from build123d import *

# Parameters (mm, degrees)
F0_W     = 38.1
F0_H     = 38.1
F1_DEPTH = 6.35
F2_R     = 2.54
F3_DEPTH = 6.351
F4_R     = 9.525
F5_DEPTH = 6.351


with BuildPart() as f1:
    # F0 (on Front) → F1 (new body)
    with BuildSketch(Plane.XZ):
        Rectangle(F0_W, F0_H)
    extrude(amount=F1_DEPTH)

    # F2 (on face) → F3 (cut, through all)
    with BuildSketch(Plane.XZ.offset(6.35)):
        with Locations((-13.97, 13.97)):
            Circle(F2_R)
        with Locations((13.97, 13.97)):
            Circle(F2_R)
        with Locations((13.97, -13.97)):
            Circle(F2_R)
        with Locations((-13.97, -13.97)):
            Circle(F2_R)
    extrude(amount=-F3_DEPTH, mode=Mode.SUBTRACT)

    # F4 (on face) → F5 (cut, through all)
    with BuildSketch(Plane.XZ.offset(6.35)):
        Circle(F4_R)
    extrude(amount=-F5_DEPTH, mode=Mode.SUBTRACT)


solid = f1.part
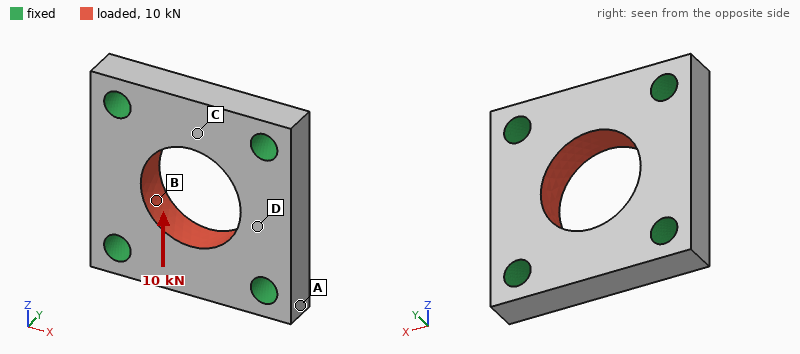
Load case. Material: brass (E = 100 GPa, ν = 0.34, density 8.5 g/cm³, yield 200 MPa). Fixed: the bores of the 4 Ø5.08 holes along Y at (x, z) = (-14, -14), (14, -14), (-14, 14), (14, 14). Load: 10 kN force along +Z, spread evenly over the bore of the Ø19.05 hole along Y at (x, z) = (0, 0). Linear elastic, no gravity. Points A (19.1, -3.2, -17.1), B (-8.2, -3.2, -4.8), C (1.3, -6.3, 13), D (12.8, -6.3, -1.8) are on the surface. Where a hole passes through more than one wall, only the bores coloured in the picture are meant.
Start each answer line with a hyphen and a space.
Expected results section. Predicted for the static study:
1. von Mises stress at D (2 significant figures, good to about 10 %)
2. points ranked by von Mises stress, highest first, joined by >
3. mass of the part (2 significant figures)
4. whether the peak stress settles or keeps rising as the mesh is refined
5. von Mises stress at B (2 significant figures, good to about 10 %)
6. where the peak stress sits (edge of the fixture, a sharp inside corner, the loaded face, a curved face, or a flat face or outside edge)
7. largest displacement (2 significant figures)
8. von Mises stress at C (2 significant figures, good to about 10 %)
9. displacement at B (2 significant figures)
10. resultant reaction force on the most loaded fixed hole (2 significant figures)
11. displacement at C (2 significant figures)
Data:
- 32 MPa
- B > D > C > A
- 59 g
- keeps rising
- 53 MPa
- edge of the fixture
- 8.2 µm
- 19 MPa
- 4.4 µm
- 2.6 kN
- 7.4 µm
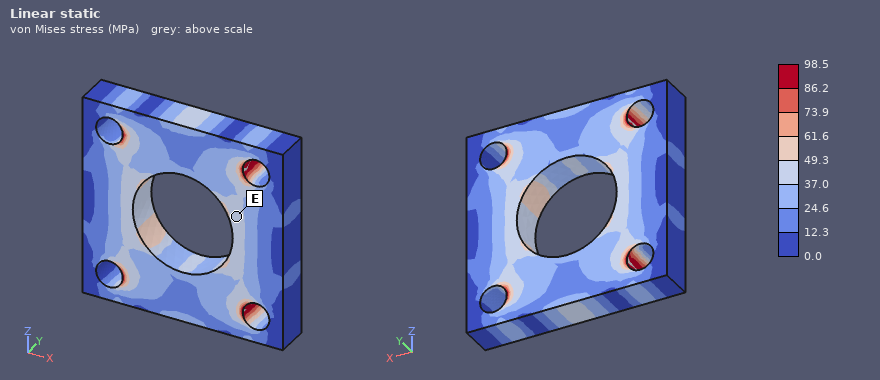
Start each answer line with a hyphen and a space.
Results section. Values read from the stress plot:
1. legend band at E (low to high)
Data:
- 37.0 to 49.3 MPa
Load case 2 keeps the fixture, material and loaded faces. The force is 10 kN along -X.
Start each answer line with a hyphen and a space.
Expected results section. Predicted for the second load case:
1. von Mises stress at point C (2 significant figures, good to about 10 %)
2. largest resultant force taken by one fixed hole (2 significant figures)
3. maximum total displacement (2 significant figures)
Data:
- 31 MPa
- 2.6 kN
- 8.2 µm
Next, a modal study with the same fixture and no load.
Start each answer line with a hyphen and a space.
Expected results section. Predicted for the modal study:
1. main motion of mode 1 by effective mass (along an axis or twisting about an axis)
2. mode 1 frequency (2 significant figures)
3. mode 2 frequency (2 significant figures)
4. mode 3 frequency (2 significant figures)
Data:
- along Y
- 25 kHz
- 27 kHz
- 27 kHz
